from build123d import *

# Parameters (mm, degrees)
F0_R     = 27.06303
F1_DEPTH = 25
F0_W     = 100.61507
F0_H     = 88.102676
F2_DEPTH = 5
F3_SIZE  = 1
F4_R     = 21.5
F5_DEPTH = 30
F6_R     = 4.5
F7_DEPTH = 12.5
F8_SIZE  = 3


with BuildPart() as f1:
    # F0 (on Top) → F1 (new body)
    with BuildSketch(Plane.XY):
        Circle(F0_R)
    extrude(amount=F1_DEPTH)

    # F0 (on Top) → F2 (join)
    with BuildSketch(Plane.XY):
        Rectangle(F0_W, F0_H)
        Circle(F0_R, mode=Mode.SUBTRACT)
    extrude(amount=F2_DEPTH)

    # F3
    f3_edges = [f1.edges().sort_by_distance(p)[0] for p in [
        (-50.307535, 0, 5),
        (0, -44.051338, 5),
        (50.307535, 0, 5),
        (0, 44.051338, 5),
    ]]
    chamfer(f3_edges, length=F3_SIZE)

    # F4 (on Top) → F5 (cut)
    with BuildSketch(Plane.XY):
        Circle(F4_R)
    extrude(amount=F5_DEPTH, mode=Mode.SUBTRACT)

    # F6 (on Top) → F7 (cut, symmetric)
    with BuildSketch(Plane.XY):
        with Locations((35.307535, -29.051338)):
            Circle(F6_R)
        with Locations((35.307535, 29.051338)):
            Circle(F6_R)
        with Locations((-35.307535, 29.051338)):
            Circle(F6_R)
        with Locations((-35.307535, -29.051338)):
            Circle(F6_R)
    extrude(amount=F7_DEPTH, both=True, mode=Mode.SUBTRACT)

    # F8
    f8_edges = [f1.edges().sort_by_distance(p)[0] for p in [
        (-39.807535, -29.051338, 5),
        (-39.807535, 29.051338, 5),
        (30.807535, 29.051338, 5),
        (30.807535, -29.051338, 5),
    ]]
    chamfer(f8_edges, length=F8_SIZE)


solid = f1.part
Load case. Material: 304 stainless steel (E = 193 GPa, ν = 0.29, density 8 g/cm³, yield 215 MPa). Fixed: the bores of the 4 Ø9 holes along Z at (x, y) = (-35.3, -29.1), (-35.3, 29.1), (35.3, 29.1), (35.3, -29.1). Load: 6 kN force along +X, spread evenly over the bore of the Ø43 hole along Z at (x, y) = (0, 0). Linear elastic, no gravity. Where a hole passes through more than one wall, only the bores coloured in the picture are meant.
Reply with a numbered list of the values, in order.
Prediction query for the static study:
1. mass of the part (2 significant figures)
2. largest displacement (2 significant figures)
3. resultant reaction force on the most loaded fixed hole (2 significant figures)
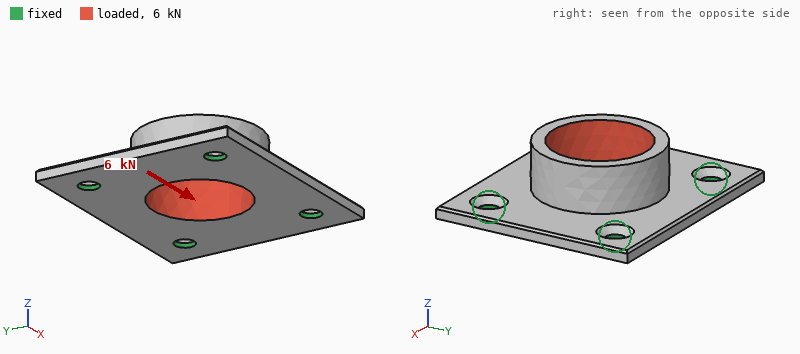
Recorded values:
1. 420 g
2. 12 µm
3. 1.7 kN
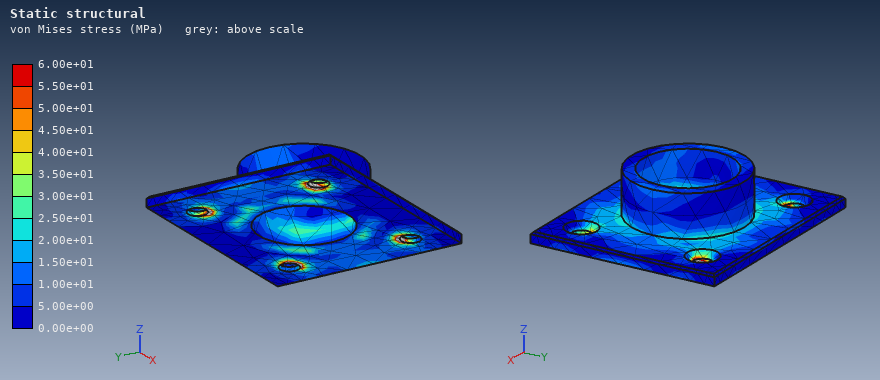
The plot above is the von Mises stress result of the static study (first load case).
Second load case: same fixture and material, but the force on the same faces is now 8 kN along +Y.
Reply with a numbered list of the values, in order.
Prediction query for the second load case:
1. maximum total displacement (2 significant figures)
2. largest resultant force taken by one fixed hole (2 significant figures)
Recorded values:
1. 24 µm
2. 2.4 kN
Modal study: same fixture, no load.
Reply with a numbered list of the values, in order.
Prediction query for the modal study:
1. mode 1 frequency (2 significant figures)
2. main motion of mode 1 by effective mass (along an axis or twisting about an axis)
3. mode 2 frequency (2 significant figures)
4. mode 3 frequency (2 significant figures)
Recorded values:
1. 4600 Hz
2. along Z
3. 4900 Hz
4. 6300 Hz
